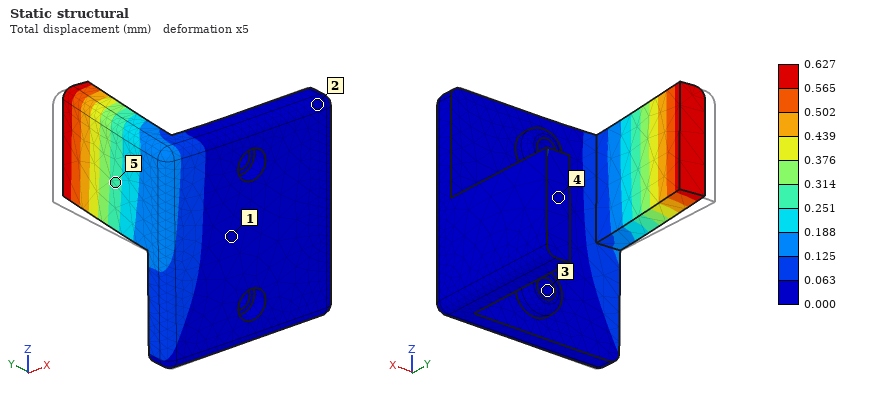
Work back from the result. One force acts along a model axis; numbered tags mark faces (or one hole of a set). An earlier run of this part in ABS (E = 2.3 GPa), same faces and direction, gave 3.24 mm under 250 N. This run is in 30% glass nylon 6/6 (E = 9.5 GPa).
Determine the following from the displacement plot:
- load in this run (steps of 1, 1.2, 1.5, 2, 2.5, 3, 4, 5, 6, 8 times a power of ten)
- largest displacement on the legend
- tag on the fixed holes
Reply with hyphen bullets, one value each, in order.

- 200 N
- 0.627 mm
- 3
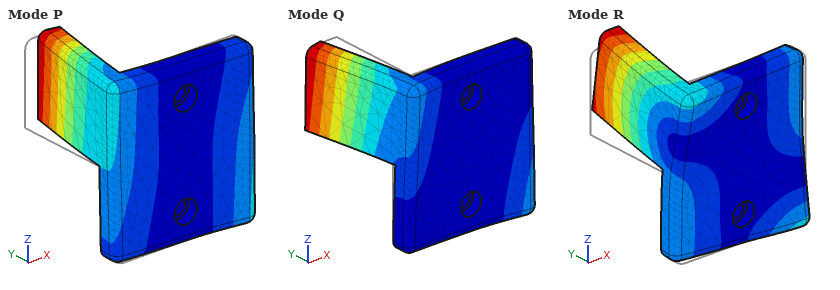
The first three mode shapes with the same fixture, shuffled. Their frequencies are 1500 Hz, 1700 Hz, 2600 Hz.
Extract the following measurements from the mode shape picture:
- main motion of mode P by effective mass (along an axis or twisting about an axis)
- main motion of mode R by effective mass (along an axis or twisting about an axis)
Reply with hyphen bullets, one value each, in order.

- along X
- twisting about Y
